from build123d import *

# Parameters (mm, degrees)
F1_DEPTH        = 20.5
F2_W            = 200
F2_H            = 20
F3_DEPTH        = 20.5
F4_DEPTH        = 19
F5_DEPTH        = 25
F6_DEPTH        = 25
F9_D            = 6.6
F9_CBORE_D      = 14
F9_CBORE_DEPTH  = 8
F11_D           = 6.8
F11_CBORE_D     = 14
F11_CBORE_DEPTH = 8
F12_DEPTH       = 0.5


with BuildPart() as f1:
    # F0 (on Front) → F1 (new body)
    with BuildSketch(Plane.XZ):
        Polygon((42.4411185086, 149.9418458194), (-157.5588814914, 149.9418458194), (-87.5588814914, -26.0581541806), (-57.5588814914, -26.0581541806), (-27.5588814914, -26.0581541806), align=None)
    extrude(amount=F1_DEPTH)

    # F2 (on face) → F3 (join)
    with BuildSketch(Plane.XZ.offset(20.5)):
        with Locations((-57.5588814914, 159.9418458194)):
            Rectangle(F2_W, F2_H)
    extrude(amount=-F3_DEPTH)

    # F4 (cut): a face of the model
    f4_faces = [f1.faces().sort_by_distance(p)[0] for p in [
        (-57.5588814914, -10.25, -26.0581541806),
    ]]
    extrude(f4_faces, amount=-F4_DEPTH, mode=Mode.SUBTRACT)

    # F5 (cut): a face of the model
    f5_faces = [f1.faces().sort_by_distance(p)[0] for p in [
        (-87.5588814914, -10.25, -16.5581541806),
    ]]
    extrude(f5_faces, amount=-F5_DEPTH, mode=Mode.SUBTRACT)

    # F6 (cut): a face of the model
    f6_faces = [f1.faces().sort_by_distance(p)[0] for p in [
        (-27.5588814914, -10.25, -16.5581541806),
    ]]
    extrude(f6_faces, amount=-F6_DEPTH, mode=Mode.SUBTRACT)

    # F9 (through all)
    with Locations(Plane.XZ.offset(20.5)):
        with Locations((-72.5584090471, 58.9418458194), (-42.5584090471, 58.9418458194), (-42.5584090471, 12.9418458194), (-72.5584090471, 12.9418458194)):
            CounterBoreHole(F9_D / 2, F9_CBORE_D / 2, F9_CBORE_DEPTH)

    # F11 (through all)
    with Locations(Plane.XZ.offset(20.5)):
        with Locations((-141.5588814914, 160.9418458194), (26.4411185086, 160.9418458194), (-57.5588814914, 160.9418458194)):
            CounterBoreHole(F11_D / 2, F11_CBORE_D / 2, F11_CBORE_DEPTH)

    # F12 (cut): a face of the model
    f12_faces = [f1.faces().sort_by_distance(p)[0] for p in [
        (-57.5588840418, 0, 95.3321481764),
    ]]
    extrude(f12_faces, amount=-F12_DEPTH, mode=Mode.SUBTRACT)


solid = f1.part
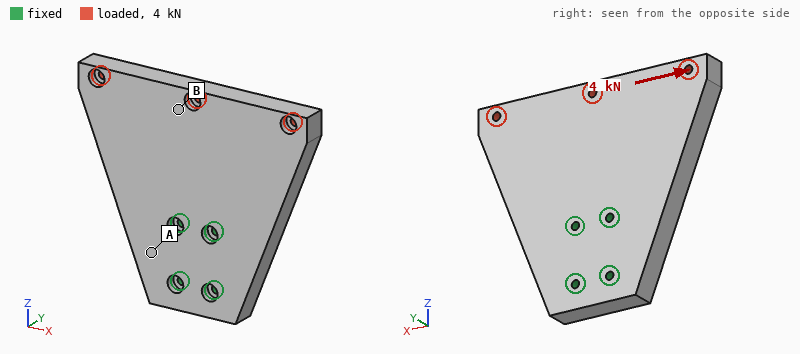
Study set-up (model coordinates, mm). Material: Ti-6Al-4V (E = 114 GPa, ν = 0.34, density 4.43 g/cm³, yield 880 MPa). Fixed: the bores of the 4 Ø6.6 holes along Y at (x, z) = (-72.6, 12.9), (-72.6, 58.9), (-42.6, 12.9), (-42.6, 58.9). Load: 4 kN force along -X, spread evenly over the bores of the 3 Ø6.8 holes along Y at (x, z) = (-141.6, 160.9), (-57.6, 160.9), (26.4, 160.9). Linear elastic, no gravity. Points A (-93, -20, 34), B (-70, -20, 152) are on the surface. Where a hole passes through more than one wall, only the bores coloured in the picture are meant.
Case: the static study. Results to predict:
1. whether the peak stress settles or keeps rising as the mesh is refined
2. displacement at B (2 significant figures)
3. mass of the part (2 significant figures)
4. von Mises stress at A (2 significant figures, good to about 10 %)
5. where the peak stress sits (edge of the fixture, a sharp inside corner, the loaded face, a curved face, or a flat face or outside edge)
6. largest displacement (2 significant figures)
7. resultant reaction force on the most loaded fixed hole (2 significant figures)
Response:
keeps rising
16 µm
2.2 kg
5.6 MPa
edge of the fixture
29 µm
5.6 kN
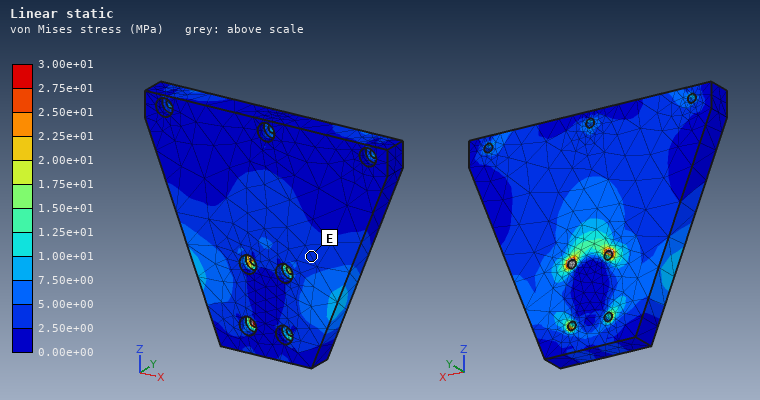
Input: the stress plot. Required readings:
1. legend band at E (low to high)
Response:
2.50e+00 to 5.00e+00 MPa
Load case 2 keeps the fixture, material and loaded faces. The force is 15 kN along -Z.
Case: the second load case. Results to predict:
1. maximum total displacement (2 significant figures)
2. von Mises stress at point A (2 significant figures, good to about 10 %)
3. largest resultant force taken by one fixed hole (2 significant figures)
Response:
39 µm
4.2 MPa
5.4 kN
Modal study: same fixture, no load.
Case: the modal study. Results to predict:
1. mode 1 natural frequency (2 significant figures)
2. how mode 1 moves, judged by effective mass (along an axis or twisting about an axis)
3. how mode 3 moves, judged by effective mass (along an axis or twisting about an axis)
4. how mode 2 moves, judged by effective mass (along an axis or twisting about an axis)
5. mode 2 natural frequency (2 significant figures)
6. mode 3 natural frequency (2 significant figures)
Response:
870 Hz
along Y
along X
twisting about Z
1200 Hz
2300 Hz
